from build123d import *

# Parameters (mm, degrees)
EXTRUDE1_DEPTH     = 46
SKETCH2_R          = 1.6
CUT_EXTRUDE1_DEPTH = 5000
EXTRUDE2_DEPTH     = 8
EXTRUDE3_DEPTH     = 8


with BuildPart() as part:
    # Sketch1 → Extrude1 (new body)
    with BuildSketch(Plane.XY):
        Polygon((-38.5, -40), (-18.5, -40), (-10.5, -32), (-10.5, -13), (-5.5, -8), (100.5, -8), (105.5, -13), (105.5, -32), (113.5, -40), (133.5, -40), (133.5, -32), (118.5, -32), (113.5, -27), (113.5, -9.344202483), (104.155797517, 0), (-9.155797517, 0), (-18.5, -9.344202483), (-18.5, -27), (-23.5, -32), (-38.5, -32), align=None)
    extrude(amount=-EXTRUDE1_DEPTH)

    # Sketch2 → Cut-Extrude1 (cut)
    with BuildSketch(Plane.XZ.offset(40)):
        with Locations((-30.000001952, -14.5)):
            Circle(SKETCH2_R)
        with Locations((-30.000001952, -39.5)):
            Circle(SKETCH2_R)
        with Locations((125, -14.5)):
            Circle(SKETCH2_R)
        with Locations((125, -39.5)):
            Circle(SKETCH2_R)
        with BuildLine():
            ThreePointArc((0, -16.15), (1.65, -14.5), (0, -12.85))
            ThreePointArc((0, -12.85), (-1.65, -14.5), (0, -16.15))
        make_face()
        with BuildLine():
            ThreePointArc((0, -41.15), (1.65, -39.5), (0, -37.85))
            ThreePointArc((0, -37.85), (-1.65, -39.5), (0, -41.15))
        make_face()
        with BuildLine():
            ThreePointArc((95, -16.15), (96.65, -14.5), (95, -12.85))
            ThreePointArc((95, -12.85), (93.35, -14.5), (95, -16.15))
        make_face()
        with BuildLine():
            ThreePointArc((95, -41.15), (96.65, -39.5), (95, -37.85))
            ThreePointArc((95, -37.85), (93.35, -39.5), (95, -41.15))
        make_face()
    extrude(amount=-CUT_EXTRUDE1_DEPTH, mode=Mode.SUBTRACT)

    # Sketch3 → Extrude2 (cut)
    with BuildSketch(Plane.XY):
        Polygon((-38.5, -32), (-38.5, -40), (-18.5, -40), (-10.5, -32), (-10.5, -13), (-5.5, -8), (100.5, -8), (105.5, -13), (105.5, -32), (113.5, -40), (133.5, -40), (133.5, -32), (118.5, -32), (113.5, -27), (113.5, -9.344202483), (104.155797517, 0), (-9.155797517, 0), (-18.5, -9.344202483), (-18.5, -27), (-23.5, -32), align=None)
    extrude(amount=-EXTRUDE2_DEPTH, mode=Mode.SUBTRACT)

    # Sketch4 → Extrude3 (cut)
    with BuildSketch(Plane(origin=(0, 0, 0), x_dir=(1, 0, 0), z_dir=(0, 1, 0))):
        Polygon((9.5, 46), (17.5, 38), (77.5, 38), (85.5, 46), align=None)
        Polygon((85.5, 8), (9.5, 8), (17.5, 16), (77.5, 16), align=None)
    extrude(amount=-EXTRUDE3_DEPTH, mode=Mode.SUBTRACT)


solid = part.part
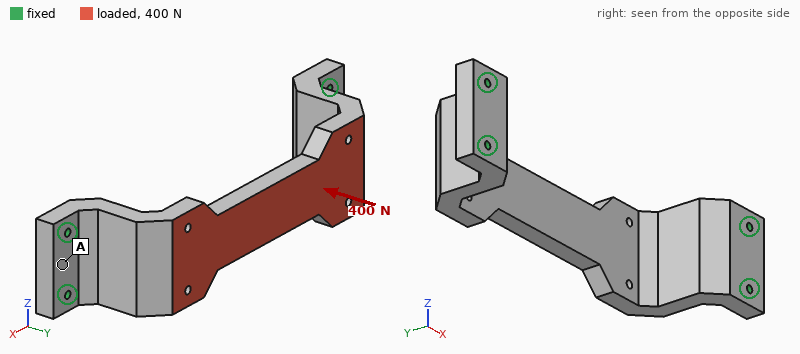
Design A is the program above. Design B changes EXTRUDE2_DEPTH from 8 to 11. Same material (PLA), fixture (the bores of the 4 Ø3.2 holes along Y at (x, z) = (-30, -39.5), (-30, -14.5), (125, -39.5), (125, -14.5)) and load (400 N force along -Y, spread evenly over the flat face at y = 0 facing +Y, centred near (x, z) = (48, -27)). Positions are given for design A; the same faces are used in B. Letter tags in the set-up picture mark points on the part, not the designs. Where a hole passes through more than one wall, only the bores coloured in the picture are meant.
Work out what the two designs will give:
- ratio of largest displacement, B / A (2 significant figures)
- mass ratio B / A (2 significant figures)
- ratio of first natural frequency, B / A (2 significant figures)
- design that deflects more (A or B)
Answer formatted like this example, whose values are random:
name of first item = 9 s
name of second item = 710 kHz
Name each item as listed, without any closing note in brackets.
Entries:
ratio of largest displacement, B / A = 1.1
mass ratio B / A = 0.94
ratio of first natural frequency, B / A = 0.99
design that deflects more = B
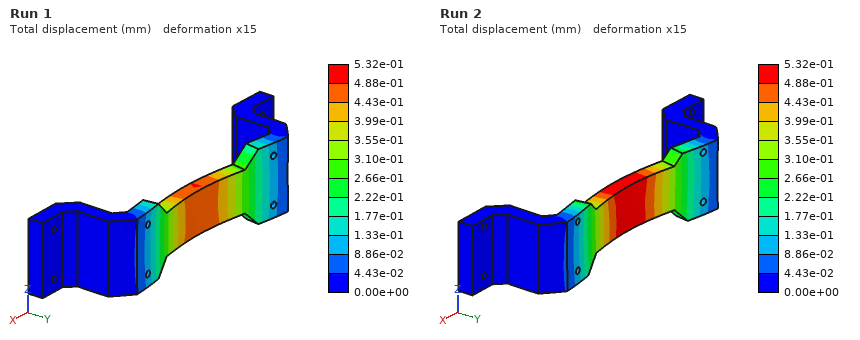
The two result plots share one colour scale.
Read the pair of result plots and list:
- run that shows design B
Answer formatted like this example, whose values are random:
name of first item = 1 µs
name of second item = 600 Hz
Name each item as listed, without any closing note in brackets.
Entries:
run that shows design B = Run 2
